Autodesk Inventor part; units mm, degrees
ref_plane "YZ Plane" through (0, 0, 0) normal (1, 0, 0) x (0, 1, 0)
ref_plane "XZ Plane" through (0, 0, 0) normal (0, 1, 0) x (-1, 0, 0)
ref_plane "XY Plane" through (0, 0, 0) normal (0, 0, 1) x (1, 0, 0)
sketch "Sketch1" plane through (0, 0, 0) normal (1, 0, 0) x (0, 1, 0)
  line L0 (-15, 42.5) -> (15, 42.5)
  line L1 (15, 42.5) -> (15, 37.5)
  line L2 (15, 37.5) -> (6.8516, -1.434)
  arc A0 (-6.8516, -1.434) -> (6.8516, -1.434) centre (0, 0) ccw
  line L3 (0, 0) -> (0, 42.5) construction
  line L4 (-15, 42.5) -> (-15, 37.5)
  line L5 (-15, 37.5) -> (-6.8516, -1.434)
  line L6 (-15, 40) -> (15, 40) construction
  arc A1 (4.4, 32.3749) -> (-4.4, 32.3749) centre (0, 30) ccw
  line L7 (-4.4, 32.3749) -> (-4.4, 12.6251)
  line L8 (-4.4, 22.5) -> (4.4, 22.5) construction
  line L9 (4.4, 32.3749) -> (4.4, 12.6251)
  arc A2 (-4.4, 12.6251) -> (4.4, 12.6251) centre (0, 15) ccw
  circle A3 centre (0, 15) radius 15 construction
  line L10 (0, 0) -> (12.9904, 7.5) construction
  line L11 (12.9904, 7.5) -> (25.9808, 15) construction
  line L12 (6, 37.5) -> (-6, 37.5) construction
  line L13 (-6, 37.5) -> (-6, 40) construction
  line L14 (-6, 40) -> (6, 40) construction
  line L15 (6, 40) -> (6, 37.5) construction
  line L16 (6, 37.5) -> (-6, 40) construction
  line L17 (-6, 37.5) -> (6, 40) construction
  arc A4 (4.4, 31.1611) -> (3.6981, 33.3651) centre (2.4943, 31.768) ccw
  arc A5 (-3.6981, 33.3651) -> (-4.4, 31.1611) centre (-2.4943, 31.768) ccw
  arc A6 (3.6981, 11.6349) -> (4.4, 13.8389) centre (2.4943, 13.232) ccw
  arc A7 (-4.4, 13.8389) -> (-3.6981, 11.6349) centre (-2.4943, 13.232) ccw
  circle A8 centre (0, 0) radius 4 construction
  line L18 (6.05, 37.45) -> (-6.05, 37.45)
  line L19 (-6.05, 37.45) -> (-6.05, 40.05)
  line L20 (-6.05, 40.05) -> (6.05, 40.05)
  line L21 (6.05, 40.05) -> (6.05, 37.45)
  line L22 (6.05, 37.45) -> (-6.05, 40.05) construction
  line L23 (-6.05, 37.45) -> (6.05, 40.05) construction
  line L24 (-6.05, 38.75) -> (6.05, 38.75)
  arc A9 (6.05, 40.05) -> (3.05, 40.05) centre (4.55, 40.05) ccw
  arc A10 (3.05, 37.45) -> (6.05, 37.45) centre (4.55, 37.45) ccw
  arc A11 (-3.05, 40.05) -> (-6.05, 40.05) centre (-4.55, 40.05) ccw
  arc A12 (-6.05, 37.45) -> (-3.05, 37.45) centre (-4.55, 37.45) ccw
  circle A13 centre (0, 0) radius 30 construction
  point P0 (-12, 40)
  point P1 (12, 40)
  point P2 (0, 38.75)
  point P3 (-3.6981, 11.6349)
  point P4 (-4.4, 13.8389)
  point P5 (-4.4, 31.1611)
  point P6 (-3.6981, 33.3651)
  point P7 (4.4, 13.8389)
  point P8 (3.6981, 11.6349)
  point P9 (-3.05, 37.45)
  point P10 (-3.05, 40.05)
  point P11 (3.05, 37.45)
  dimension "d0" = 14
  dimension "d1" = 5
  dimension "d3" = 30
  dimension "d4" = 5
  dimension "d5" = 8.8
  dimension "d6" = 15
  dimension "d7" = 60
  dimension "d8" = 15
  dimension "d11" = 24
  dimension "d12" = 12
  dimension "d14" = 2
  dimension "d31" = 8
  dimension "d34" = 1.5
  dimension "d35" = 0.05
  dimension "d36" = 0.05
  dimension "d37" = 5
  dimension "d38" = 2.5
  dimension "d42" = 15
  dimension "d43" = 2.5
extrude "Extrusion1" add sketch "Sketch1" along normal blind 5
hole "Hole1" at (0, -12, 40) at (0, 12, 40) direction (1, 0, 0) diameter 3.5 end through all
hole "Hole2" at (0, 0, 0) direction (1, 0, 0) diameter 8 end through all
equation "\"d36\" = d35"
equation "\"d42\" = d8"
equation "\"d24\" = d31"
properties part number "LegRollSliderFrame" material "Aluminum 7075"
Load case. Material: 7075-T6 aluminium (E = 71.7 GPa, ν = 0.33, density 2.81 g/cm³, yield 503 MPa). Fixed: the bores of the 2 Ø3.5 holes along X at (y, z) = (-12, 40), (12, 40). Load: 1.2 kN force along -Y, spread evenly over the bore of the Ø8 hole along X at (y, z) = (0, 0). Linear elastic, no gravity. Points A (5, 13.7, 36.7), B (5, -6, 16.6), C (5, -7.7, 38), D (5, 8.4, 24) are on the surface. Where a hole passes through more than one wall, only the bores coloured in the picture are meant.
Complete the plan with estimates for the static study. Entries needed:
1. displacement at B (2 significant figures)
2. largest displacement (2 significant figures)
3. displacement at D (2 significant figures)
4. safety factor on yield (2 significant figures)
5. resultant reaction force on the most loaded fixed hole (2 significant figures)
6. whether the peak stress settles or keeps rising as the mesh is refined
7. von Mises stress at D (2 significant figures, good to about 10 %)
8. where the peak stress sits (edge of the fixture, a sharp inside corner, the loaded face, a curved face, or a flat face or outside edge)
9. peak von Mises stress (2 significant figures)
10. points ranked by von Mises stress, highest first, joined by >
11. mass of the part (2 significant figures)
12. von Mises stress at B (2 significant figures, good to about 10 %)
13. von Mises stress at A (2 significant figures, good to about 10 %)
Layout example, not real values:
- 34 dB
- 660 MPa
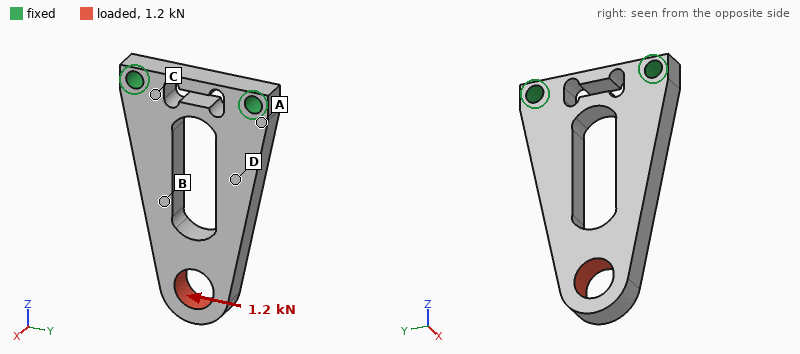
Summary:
- 0.085 mm
- 0.14 mm
- 0.045 mm
- 1.8
- 1.7 kN
- settles
- 49 MPa
- a curved face
- 280 MPa
- A > B > D > C
- 10 g
- 73 MPa
- 93 MPa
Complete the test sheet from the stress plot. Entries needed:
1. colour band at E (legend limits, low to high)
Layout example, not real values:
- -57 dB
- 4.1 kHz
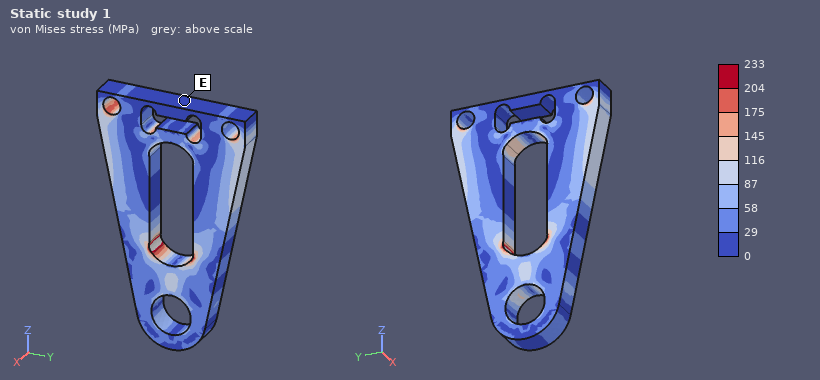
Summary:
- 0 to 29 MPa
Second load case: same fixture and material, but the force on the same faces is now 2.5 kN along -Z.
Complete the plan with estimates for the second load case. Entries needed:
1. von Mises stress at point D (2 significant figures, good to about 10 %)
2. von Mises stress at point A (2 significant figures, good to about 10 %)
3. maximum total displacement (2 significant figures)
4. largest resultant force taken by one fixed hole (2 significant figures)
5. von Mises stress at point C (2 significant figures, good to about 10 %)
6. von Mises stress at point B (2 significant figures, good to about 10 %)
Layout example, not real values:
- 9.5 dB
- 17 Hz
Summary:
- 33 MPa
- 25 MPa
- 28 µm
- 1.3 kN
- 20 MPa
- 47 MPa
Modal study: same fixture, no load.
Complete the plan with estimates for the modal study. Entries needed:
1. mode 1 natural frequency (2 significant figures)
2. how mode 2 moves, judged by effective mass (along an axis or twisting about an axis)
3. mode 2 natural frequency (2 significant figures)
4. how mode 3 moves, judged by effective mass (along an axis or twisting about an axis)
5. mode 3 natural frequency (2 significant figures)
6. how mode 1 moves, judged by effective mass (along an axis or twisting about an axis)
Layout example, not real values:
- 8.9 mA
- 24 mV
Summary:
- 2400 Hz
- along Y
- 7600 Hz
- twisting about Z
- 9100 Hz
- along X
